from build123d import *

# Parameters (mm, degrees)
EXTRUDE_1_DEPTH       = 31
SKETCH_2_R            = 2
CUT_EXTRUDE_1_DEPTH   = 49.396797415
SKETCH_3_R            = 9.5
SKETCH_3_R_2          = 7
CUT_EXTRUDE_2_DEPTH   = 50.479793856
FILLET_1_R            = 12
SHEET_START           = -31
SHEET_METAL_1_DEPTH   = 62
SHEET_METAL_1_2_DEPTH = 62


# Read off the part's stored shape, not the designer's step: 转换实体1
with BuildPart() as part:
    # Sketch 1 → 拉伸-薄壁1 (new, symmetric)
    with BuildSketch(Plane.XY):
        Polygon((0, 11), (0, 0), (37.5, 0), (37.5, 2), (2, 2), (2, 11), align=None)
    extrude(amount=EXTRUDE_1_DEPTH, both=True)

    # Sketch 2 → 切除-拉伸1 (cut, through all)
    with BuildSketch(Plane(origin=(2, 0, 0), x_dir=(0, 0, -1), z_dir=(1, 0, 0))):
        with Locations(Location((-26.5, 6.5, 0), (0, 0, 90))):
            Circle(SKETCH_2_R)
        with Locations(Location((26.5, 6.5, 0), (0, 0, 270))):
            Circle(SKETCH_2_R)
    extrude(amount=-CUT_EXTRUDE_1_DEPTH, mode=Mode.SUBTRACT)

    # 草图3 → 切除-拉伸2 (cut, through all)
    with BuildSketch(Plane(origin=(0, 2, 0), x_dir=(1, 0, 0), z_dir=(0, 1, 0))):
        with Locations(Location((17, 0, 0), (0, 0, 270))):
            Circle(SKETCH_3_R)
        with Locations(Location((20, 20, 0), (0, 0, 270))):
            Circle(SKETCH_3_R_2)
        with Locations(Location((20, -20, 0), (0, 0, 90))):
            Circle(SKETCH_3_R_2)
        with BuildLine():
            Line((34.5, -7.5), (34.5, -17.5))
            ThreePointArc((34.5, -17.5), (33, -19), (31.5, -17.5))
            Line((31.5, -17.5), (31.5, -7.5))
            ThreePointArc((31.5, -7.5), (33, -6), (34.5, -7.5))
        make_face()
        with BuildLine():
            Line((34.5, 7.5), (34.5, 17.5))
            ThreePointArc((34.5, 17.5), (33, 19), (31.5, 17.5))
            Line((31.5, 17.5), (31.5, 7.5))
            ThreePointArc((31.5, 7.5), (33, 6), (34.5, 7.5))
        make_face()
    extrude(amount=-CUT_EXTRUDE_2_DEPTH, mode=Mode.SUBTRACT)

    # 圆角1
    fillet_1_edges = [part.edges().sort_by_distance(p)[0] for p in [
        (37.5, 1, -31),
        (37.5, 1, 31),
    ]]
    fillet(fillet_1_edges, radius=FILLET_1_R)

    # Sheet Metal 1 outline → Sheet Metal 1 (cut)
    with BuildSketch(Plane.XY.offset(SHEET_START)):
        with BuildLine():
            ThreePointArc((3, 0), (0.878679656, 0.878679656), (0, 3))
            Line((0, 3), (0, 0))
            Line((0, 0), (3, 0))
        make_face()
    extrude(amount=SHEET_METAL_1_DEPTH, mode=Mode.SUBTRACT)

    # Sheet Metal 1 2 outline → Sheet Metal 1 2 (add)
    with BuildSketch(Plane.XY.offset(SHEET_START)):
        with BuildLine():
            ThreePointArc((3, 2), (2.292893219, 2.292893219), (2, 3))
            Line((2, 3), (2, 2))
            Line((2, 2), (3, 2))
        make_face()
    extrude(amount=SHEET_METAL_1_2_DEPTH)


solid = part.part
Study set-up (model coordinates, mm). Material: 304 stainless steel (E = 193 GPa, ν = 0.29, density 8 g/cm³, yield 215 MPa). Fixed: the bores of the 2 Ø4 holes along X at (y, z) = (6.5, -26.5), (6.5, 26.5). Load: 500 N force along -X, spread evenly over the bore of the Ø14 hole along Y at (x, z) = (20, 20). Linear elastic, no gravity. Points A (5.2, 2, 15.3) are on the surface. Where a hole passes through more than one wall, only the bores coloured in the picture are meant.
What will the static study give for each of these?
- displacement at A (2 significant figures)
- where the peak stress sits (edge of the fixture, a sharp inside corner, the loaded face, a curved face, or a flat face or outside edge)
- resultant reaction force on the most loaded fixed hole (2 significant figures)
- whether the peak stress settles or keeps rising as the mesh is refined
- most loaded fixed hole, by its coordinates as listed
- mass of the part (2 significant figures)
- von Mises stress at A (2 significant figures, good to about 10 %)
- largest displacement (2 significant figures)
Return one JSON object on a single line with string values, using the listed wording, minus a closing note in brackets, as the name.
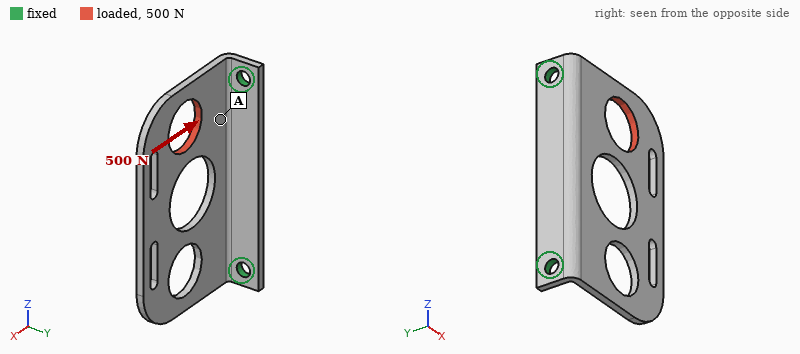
{"displacement at A": "11 µm", "where the peak stress sits": "edge of the fixture", "resultant reaction force on the most loaded fixed hole": "440 N", "whether the peak stress settles or keeps rising as the mesh is refined": "keeps rising", "most loaded fixed hole, by its coordinates as listed": "(6.5, 26.5)", "mass of the part": "33 g", "von Mises stress at A": "18 MPa", "largest displacement": "64 µm"}
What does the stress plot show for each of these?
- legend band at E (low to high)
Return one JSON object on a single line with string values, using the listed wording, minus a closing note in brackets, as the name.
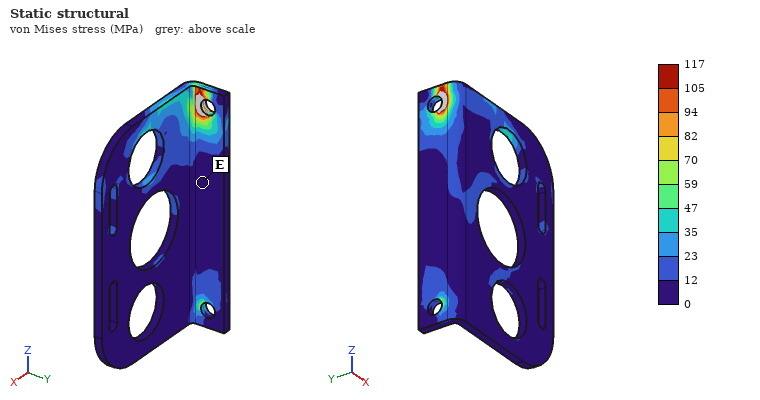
{"legend band at E": "0 to 12 MPa"}
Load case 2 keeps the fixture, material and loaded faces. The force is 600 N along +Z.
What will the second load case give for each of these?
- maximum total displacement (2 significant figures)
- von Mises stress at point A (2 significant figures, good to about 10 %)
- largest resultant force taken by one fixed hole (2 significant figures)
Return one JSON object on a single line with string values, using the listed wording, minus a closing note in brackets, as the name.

{"maximum total displacement": "23 µm", "von Mises stress at point A": "22 MPa", "largest resultant force taken by one fixed hole": "390 N"}
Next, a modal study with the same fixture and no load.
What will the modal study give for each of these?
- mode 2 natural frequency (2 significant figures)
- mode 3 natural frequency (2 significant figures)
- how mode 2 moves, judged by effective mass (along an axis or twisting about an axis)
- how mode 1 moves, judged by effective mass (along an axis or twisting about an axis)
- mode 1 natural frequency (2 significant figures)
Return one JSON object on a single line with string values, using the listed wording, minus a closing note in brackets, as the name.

{"mode 2 natural frequency": "1900 Hz", "mode 3 natural frequency": "3900 Hz", "how mode 2 moves, judged by effective mass": "twisting about X", "how mode 1 moves, judged by effective mass": "along Y", "mode 1 natural frequency": "890 Hz"}
